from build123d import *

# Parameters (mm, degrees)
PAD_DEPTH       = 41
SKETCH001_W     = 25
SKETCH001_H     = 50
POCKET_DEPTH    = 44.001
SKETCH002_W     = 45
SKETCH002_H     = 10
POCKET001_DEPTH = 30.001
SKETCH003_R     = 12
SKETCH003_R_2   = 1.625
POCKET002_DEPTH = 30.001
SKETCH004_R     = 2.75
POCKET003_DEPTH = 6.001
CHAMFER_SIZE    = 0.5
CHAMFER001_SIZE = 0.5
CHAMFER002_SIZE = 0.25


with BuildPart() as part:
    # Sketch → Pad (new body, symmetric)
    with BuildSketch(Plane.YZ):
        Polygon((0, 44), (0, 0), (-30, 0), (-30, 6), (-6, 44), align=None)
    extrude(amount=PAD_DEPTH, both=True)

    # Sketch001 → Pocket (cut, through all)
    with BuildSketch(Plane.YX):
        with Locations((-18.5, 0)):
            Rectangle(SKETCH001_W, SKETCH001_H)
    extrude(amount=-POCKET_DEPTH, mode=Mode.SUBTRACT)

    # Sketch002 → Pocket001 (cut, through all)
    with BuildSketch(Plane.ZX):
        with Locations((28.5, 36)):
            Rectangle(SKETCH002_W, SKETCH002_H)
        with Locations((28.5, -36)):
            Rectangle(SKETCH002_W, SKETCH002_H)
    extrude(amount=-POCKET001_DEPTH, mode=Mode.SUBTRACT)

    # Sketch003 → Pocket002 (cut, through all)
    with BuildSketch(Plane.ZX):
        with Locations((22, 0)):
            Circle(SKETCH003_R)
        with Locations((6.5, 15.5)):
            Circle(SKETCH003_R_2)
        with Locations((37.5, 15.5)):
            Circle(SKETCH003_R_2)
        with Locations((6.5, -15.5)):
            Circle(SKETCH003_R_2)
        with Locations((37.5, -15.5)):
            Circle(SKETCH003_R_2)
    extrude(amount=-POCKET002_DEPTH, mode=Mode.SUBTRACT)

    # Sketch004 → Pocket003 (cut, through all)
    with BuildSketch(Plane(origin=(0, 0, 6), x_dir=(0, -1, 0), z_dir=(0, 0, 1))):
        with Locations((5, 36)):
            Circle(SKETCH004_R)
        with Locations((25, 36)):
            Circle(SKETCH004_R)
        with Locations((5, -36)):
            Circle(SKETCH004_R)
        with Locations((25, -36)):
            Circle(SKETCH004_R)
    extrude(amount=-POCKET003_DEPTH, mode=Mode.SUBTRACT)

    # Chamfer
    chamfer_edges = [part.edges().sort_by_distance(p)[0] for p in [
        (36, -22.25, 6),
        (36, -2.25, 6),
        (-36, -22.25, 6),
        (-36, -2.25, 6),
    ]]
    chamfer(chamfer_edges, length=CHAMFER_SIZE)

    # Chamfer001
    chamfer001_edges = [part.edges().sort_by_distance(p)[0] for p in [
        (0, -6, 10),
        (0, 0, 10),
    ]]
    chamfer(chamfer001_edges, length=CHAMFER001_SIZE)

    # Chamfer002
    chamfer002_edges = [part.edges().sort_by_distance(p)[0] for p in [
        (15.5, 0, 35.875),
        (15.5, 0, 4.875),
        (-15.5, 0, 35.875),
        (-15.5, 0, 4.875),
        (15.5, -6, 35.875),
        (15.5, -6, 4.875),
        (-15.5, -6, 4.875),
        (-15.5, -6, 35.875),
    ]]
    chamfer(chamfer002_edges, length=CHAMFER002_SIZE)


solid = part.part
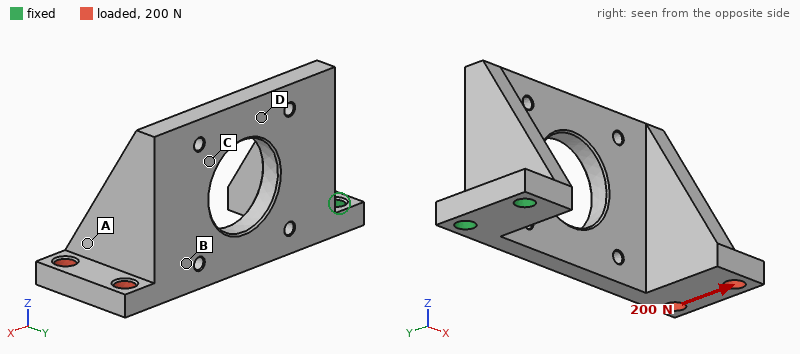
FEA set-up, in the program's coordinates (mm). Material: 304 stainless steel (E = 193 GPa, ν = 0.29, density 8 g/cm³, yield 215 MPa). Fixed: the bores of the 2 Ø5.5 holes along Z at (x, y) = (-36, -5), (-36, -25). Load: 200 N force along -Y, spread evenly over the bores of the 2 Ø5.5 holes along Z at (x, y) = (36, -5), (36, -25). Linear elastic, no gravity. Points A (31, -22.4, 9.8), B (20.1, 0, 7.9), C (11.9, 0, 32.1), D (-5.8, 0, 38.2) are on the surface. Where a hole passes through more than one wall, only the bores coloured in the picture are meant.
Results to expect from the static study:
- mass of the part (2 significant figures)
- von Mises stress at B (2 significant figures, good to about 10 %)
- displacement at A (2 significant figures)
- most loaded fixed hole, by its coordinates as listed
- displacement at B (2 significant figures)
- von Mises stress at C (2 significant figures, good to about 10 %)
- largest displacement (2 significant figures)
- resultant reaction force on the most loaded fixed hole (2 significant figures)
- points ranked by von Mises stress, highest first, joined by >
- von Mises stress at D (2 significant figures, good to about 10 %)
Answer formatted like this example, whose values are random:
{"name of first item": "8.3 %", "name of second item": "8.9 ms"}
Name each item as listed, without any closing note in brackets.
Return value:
{"mass of the part": "190 g", "von Mises stress at B": "20 MPa", "displacement at A": "0.23 mm", "most loaded fixed hole, by its coordinates as listed": "(-36, -25)", "displacement at B": "0.16 mm", "von Mises stress at C": "38 MPa", "largest displacement": "0.30 mm", "resultant reaction force on the most loaded fixed hole": "730 N", "points ranked by von Mises stress, highest first, joined by >": "D > C > B > A", "von Mises stress at D": "55 MPa"}
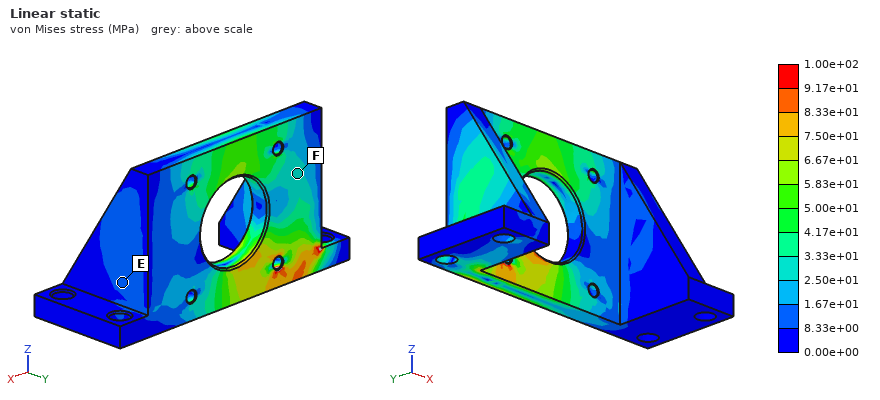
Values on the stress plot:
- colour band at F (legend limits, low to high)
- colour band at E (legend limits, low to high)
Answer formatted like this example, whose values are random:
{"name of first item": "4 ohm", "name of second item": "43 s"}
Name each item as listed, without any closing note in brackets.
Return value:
{"colour band at F": "2.50e+01 to 3.33e+01 MPa", "colour band at E": "8.33e+00 to 1.67e+01 MPa"}
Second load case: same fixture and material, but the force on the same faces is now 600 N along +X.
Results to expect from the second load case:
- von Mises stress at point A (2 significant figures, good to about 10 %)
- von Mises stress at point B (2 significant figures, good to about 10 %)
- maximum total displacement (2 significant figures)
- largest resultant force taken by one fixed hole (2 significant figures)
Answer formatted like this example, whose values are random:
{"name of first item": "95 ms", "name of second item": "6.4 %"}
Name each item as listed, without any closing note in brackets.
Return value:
{"von Mises stress at point A": "10 MPa", "von Mises stress at point B": "30 MPa", "maximum total displacement": "0.26 mm", "largest resultant force taken by one fixed hole": "350 N"}
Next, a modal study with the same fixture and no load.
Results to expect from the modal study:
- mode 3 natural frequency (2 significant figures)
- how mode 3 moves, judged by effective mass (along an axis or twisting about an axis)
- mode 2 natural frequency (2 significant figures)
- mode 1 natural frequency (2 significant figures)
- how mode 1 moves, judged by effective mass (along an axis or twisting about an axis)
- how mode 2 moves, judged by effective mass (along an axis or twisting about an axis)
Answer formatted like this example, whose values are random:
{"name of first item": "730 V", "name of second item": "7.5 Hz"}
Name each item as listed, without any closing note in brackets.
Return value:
{"mode 3 natural frequency": "2000 Hz", "how mode 3 moves, judged by effective mass": "twisting about X", "mode 2 natural frequency": "750 Hz", "mode 1 natural frequency": "610 Hz", "how mode 1 moves, judged by effective mass": "along Y", "how mode 2 moves, judged by effective mass": "along Z"}
